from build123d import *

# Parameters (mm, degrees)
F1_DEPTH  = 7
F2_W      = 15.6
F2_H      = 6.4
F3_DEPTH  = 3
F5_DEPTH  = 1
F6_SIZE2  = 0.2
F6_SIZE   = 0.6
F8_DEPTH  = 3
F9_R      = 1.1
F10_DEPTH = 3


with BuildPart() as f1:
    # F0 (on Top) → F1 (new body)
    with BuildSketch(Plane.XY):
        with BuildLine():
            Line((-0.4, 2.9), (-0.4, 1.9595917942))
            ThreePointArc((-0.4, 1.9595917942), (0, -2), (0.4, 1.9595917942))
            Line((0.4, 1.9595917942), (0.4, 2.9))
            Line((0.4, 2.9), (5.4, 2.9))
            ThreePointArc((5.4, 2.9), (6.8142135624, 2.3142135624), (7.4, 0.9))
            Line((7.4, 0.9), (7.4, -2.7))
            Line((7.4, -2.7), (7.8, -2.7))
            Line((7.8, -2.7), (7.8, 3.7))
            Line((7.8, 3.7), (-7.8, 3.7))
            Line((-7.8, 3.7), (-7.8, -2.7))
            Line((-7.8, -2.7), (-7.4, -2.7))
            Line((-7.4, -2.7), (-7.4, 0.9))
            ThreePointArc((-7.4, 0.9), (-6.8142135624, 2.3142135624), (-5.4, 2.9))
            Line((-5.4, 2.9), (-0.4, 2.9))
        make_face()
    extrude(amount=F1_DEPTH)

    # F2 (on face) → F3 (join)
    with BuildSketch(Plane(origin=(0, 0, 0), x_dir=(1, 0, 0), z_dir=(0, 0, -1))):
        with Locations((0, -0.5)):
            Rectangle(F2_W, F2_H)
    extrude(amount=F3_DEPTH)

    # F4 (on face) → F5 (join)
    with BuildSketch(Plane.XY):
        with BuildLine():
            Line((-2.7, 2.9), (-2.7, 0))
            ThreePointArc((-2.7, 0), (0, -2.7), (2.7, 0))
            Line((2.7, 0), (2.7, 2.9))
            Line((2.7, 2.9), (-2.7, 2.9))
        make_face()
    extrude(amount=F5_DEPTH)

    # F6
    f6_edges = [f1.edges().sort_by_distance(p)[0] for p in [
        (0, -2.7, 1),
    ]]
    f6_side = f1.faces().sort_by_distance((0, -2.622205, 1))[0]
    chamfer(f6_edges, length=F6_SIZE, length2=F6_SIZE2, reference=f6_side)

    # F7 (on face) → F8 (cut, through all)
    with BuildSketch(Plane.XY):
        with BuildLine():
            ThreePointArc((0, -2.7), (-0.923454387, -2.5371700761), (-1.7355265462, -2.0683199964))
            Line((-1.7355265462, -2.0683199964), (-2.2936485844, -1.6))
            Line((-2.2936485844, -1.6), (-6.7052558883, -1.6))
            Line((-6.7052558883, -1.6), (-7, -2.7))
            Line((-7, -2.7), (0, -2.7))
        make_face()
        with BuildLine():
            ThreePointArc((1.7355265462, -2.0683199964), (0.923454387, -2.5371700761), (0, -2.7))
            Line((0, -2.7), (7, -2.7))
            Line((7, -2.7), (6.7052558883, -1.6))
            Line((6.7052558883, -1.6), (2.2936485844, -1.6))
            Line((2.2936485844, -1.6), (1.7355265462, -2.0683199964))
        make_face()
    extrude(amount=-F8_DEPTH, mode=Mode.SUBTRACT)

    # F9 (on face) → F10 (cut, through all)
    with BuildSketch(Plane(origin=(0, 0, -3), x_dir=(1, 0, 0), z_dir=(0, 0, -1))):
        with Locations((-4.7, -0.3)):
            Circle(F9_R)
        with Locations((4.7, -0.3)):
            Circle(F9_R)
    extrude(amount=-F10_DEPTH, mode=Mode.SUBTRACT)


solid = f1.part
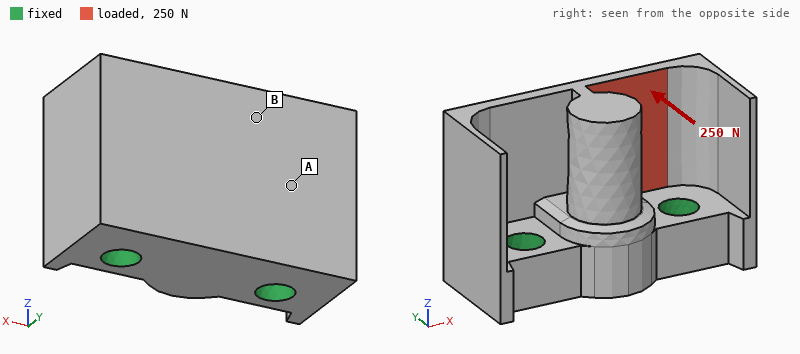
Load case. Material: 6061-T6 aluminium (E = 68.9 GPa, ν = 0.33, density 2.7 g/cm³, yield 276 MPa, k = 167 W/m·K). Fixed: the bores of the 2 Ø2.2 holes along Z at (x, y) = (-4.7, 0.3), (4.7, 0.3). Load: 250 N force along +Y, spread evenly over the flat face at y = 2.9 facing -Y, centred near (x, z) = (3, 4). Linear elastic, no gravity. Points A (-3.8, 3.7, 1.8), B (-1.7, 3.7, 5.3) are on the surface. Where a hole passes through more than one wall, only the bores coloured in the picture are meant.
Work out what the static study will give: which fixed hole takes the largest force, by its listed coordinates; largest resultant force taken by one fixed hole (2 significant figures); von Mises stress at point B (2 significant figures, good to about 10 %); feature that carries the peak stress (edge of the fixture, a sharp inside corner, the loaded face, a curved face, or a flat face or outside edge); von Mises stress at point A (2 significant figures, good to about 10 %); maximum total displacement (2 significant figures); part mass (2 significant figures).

(4.7, 0.3)
200 N
42 MPa
a flat face or outside edge
15 MPa
48 µm
1.3 g
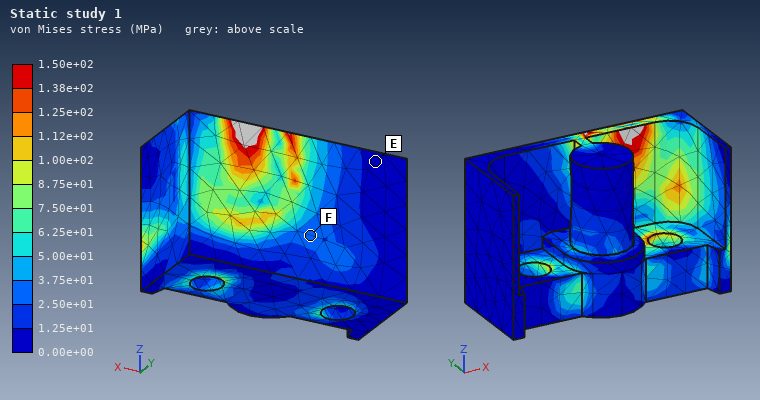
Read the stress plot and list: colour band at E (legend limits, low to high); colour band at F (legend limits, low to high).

0.00e+00 to 1.25e+01 MPa
2.50e+01 to 3.75e+01 MPa
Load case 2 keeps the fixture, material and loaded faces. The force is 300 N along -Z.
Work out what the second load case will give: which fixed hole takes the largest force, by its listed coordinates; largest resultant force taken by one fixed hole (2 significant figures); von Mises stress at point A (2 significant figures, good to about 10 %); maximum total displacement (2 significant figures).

(4.7, 0.3)
230 N
10.0 MPa
6.9 µm
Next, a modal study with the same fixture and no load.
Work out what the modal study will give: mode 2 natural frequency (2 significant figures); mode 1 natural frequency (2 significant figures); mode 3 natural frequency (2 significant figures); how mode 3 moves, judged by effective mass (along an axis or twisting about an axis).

21 kHz
21 kHz
33 kHz
along Y
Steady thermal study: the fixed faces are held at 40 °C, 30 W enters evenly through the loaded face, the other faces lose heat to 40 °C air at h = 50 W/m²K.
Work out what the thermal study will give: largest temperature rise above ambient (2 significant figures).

71 K
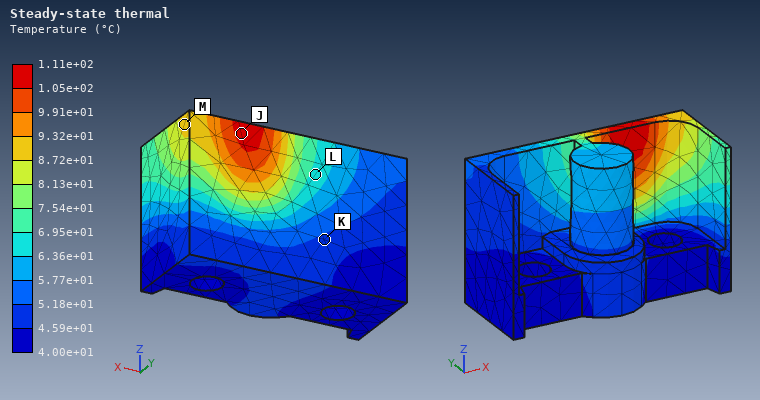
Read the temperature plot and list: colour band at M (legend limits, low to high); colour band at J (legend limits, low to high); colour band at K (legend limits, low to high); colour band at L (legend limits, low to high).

8.72e+01 to 9.32e+01 °C
1.05e+02 to 1.11e+02 °C
4.59e+01 to 5.18e+01 °C
6.36e+01 to 6.95e+01 °C
